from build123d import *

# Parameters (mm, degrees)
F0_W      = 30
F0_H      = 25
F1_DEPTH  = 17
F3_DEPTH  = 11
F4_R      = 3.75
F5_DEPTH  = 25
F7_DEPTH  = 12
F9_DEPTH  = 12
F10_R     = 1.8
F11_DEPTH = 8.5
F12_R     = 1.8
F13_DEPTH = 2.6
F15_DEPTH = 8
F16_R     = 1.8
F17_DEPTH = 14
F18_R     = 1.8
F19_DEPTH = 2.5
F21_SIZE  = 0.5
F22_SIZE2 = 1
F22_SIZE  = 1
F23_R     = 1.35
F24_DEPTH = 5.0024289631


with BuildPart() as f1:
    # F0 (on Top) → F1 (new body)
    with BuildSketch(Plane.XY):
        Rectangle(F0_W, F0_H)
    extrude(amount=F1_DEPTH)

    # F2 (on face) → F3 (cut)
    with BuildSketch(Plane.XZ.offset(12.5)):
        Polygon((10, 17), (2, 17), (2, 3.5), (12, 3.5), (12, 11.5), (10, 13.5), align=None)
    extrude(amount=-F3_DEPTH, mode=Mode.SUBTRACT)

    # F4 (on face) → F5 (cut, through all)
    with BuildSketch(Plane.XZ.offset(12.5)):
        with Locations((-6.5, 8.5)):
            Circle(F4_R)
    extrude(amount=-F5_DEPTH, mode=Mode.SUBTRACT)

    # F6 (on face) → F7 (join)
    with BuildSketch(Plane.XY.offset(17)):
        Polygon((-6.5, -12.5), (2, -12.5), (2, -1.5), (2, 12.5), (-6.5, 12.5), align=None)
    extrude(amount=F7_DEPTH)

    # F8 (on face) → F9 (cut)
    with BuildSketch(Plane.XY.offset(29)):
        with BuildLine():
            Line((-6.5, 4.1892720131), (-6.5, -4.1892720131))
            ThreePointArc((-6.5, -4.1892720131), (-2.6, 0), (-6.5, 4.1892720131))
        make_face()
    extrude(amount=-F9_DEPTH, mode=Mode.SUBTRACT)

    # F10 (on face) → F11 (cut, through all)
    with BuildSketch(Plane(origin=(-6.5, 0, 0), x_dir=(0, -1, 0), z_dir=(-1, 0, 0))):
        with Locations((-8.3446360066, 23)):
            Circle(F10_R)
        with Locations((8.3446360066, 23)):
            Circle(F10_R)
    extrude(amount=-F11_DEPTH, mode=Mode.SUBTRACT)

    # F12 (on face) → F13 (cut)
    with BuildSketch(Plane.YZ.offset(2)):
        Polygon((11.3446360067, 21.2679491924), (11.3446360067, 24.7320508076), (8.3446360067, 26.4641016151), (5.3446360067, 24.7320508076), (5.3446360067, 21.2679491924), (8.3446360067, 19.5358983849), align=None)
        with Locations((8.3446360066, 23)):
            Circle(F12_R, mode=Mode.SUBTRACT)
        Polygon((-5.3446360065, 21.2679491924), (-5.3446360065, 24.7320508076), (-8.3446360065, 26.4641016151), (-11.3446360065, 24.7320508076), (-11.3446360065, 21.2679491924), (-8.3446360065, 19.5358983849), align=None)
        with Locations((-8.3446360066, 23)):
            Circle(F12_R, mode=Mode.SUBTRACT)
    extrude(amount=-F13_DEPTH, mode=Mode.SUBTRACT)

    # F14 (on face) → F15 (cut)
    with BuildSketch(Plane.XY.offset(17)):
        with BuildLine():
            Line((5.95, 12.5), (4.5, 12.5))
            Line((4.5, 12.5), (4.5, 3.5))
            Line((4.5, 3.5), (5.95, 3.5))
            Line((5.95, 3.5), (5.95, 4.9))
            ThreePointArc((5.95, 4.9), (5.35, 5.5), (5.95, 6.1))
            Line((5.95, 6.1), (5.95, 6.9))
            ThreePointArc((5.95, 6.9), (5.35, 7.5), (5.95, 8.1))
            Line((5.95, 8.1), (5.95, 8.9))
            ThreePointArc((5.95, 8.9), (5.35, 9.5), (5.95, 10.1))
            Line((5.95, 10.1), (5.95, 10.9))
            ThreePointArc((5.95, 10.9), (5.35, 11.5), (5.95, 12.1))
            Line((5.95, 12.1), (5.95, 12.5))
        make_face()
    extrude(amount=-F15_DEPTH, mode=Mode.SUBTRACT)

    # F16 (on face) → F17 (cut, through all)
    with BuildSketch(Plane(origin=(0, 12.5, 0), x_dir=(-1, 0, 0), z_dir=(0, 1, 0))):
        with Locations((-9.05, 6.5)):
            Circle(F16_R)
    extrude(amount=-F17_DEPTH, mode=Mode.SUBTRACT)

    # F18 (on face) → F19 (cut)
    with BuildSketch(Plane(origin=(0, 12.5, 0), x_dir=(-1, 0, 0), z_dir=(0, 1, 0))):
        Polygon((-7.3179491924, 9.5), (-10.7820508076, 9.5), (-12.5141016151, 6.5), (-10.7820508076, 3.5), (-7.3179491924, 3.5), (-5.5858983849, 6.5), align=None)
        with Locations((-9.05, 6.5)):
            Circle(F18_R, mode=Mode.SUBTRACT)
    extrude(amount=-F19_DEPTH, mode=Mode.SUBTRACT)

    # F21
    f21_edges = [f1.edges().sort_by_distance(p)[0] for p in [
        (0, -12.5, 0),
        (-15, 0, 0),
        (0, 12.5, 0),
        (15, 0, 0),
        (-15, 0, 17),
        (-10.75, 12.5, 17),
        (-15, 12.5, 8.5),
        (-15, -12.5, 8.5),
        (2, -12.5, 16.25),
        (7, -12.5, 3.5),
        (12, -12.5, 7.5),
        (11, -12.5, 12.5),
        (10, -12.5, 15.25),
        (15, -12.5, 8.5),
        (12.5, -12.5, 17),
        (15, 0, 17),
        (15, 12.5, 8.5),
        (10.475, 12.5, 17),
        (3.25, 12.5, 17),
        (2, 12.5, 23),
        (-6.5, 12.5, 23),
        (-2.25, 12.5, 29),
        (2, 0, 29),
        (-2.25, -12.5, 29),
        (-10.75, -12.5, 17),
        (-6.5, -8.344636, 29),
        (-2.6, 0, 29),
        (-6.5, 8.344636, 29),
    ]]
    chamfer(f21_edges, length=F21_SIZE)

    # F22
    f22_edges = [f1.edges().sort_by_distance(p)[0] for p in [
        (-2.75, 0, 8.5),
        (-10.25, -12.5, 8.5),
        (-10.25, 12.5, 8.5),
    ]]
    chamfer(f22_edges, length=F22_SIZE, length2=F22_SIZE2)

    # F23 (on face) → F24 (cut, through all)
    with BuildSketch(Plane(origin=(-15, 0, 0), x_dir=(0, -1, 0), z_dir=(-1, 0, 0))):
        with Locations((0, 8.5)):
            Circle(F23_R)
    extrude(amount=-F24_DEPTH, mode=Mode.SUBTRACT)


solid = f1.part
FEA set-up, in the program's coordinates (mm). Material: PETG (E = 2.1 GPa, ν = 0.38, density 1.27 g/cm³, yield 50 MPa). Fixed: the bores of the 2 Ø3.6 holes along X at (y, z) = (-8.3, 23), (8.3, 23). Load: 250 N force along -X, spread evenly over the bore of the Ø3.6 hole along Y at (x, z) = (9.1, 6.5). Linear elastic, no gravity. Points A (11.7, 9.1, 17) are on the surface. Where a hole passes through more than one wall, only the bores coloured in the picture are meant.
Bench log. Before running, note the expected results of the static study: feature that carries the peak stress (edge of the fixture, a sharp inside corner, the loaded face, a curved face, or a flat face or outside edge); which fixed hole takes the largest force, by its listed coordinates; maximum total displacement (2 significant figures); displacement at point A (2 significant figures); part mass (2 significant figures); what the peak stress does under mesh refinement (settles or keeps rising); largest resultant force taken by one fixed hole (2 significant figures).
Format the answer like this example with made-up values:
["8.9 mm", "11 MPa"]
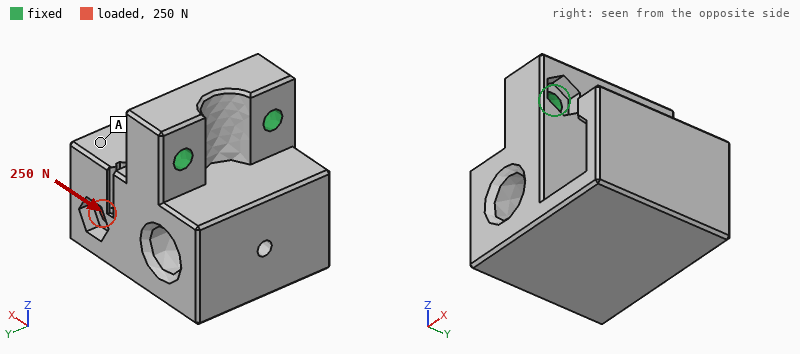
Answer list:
["edge of the fixture", "(8.3, 23)", "0.58 mm", "0.32 mm", "15 g", "keeps rising", "180 N"]
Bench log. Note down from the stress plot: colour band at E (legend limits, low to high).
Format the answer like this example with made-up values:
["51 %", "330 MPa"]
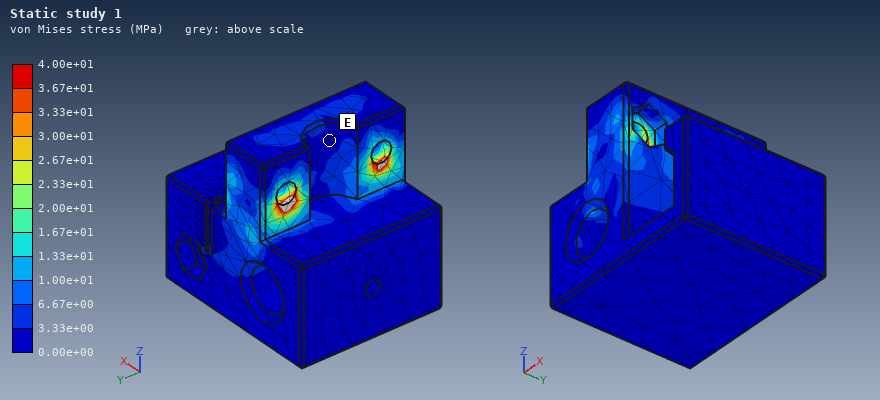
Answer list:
["0.00e+00 to 3.33e+00 MPa"]
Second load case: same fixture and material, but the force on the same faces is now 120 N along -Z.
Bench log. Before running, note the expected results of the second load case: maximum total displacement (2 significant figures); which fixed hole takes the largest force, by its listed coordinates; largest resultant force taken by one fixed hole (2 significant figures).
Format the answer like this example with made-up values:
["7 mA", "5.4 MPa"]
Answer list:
["0.26 mm", "(8.3, 23)", "91 N"]
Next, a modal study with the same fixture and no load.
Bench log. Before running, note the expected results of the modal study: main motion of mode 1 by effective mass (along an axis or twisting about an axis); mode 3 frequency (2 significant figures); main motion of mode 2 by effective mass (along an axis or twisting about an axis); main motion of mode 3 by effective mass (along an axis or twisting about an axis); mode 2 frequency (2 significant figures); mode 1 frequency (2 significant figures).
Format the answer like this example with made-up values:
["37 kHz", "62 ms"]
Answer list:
["along X", "3300 Hz", "along Y", "along Y", "2600 Hz", "1100 Hz"]
